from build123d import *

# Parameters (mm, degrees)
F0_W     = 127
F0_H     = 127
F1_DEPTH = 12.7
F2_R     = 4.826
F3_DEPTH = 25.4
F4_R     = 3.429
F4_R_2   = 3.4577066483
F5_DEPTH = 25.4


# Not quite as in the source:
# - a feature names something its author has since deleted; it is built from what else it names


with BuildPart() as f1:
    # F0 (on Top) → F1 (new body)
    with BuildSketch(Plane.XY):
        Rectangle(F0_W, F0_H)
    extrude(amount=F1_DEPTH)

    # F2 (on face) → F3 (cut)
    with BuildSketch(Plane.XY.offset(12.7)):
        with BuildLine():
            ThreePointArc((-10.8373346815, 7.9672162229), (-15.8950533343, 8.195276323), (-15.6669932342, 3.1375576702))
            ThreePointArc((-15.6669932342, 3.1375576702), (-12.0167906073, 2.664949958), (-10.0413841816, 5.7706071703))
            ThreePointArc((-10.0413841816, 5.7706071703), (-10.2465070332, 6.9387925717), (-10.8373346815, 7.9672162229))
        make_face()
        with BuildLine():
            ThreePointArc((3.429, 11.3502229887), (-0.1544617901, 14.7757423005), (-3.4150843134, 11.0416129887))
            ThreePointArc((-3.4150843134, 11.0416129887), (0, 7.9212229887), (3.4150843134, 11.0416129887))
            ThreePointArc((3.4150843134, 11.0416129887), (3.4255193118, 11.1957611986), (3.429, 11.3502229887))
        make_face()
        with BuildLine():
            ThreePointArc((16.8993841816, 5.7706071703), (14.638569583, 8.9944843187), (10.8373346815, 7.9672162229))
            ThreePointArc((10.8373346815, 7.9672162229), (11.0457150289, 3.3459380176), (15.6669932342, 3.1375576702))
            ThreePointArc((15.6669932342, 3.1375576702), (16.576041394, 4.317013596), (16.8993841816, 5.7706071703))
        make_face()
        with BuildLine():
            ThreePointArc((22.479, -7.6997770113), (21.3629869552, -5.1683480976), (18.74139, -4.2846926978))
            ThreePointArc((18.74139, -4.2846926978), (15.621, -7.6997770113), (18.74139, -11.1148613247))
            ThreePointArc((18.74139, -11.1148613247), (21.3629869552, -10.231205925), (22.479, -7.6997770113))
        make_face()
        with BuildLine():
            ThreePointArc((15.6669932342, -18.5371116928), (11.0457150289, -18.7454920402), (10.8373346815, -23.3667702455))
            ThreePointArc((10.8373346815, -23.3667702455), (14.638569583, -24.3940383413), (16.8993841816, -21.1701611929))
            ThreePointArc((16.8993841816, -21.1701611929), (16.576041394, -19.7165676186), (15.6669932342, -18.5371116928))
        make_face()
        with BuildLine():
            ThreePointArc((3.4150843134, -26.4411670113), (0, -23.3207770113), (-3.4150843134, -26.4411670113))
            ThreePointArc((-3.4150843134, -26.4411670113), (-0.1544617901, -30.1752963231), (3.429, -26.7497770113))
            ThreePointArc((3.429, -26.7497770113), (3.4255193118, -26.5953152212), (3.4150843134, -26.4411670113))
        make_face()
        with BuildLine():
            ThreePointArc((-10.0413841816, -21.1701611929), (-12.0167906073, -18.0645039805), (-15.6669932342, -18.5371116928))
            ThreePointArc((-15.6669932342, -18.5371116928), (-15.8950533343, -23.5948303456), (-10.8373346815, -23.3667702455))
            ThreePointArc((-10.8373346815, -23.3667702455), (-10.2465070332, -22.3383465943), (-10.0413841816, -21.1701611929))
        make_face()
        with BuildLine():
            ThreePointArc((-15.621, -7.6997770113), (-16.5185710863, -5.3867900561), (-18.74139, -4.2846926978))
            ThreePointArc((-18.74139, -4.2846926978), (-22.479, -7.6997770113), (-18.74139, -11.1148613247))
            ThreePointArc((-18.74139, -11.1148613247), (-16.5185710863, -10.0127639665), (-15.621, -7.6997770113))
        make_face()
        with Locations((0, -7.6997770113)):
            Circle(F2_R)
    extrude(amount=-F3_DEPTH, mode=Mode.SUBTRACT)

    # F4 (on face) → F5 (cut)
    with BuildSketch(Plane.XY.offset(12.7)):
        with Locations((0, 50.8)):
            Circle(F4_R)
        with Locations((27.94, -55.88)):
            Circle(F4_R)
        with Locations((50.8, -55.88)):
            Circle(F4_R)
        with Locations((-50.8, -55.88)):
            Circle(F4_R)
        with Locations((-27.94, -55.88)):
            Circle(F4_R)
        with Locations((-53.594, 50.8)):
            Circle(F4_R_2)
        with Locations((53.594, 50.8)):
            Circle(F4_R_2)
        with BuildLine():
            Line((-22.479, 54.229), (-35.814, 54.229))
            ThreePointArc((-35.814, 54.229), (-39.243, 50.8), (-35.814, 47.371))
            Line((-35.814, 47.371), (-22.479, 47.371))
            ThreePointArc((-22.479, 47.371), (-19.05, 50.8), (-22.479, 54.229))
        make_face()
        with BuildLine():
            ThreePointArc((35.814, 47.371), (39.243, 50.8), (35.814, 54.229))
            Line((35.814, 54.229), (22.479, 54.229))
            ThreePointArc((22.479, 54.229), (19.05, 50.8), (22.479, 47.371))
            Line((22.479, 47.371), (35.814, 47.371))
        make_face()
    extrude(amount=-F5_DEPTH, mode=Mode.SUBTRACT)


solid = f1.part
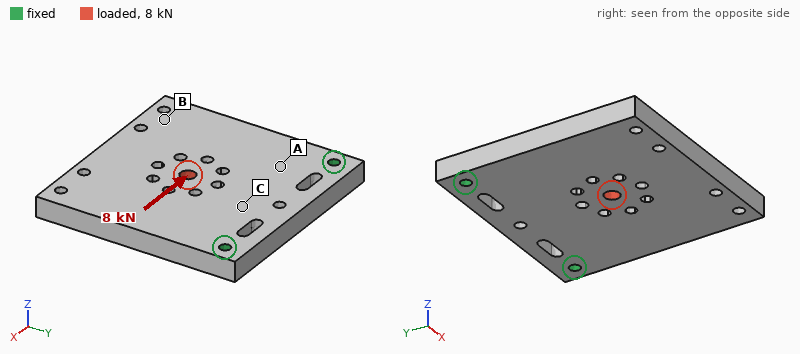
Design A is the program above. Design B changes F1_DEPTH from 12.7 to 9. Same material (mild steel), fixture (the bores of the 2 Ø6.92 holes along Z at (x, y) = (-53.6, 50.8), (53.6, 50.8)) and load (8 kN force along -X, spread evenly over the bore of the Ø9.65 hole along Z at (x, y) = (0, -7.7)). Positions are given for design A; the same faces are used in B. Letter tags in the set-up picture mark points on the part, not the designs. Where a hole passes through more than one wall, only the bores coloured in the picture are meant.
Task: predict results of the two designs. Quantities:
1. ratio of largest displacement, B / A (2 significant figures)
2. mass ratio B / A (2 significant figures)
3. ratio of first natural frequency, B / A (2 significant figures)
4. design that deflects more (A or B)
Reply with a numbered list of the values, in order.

1. 1.4
2. 0.71
3. 0.73
4. B
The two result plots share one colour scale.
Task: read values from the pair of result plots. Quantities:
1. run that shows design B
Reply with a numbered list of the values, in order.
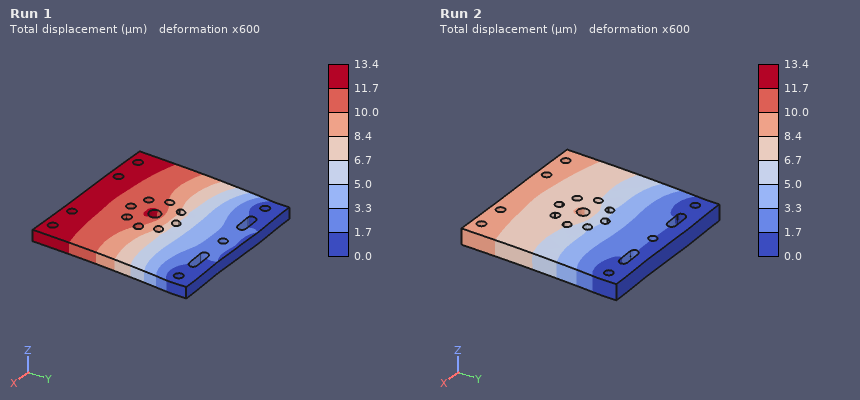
1. Run 1
